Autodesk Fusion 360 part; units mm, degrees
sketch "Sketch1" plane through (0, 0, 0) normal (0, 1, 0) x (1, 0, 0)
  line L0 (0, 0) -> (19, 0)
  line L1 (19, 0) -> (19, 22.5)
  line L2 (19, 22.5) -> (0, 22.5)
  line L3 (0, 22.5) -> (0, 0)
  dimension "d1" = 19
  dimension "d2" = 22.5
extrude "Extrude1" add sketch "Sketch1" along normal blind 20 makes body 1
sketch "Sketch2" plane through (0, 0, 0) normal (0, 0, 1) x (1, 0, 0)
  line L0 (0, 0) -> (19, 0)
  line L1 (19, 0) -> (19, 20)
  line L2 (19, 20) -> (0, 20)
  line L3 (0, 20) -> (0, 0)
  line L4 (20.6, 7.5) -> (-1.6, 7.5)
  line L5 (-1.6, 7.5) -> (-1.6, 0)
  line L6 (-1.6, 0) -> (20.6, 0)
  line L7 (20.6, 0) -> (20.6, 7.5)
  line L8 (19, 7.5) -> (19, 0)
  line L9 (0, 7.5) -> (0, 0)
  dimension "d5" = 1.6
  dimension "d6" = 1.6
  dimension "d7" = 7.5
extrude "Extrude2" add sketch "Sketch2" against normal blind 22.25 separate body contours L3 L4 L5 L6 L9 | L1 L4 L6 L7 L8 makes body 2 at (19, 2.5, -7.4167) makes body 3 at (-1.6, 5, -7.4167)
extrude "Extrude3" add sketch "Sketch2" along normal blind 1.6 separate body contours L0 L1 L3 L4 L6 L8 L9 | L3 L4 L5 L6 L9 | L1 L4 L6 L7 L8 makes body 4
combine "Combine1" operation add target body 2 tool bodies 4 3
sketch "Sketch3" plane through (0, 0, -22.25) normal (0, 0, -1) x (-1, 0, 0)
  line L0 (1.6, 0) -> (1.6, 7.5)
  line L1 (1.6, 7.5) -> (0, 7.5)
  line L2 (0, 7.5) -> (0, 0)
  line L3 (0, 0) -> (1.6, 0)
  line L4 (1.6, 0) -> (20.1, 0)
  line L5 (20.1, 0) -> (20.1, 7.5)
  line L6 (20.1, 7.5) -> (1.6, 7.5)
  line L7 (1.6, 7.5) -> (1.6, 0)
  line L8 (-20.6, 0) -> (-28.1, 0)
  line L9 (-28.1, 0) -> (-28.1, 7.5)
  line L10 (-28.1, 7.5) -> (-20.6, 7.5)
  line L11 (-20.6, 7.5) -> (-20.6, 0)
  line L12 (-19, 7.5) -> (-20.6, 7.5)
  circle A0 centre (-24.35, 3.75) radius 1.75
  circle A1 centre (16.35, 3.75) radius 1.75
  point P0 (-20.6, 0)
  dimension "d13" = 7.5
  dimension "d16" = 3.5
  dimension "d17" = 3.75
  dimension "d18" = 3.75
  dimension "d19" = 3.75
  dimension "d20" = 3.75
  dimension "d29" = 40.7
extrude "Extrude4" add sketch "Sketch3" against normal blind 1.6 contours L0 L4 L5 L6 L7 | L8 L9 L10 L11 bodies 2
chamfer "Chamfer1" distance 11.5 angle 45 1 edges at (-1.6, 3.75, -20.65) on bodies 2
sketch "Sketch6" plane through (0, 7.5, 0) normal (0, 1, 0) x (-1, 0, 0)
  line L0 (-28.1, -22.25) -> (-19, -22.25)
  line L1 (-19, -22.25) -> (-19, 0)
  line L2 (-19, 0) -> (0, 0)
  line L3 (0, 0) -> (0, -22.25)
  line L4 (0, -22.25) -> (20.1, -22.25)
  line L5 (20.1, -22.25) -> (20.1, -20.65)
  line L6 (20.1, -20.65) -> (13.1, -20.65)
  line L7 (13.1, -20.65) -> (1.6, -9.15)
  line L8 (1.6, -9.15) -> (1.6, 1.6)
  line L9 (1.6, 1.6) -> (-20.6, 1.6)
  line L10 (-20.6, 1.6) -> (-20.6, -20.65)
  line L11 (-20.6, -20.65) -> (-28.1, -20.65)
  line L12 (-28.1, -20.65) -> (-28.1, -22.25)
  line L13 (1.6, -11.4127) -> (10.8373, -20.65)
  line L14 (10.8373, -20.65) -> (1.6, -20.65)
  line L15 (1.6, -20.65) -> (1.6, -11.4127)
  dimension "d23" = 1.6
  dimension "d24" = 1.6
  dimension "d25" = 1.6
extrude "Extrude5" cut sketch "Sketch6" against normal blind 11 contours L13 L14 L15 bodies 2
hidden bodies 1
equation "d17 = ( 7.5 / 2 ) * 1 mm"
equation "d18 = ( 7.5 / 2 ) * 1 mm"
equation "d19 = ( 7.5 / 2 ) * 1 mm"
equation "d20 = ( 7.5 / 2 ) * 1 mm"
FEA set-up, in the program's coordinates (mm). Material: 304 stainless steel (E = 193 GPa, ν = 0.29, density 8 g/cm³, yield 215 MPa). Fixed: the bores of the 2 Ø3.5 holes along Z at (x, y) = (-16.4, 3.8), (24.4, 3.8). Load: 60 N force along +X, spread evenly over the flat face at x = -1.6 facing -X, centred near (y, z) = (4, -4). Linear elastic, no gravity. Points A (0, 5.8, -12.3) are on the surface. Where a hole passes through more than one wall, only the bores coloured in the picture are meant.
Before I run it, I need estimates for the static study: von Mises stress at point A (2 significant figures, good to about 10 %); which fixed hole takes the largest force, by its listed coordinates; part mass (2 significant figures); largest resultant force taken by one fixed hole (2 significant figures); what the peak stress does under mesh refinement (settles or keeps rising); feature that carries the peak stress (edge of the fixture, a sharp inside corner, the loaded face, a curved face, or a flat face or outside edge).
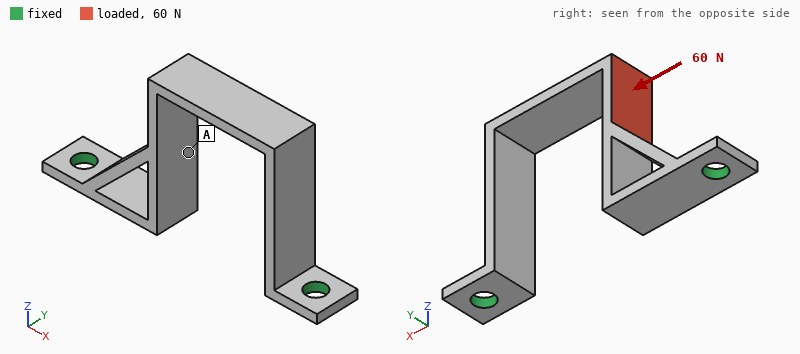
9.7 MPa
(-16.4, 3.8)
10 g
47 N
keeps rising
edge of the fixture
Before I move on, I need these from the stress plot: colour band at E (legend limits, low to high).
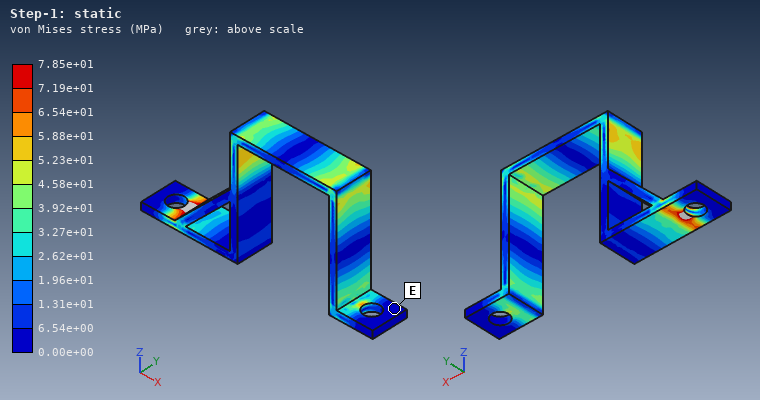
0.00e+00 to 6.54e+00 MPa
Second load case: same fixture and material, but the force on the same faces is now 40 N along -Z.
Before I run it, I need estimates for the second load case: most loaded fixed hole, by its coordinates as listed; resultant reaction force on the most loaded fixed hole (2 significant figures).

(-16.4, 3.8)
34 N
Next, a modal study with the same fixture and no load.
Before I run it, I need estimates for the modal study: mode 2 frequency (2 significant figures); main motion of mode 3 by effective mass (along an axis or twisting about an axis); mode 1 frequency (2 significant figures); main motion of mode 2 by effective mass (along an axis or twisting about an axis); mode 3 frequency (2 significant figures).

2900 Hz
twisting about Z
2500 Hz
along Y
5100 Hz
